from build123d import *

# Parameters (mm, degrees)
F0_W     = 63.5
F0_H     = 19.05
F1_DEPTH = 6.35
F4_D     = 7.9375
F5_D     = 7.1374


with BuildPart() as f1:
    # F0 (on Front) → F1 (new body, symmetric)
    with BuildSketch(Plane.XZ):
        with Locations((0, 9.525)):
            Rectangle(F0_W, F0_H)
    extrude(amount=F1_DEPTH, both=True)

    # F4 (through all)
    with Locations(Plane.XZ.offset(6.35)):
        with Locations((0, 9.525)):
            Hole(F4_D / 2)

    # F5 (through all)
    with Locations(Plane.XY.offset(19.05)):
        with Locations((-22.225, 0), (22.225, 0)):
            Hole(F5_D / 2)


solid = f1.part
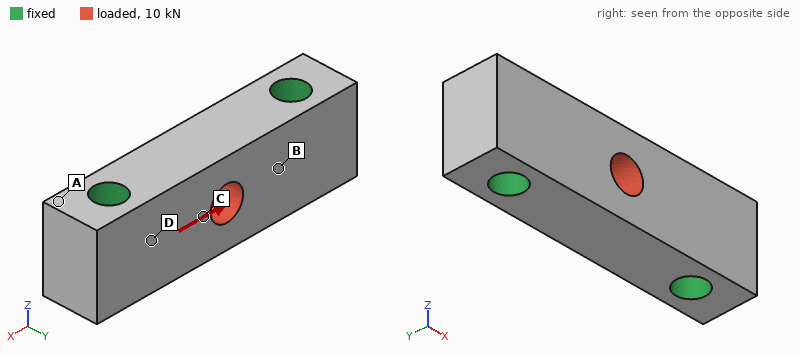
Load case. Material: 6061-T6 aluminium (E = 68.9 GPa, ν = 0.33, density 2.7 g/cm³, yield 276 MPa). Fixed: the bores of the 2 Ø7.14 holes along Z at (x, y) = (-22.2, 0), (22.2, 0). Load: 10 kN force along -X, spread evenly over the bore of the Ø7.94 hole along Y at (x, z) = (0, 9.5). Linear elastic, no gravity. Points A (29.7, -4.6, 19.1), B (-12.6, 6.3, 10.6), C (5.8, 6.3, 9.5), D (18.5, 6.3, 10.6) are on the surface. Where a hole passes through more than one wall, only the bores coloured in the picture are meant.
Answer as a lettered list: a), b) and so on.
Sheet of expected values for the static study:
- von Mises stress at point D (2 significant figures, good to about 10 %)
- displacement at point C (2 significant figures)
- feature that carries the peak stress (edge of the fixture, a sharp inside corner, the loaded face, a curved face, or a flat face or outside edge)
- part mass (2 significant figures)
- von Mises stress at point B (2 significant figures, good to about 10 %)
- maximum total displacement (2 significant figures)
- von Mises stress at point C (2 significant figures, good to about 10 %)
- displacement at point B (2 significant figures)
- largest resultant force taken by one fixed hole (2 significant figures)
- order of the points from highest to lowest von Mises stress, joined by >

a) 11 MPa
b) 5.2 µm
c) the loaded face
d) 36 g
e) 23 MPa
f) 6.8 µm
g) 34 MPa
h) 2.5 µm
i) 5.0 kN
j) C > B > D > A
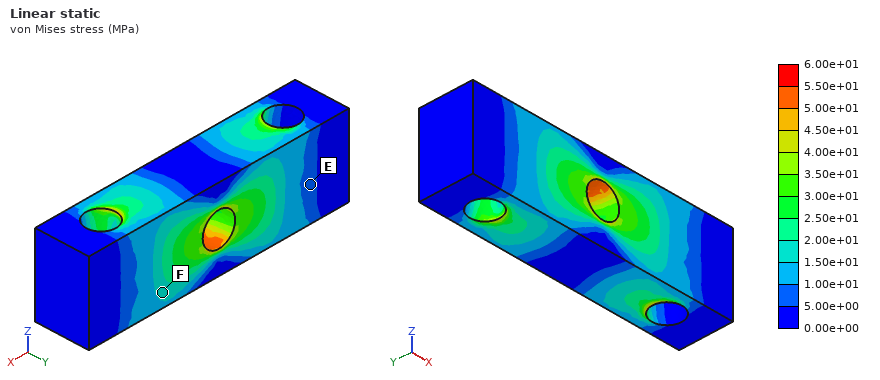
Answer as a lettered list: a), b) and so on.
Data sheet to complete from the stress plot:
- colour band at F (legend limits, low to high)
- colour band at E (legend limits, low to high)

a) 1.50e+01 to 2.00e+01 MPa
b) 5.00e+00 to 1.00e+01 MPa
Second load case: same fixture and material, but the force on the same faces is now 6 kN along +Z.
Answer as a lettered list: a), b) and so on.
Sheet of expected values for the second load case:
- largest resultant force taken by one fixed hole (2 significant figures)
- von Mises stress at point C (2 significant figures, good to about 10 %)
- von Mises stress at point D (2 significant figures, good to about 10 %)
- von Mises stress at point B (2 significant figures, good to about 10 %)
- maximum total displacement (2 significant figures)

a) 3.0 kN
b) 36 MPa
c) 15 MPa
d) 31 MPa
e) 15 µm
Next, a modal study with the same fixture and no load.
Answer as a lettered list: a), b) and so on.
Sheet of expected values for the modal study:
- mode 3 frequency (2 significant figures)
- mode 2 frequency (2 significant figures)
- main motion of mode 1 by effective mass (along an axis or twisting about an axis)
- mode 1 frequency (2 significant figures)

a) 35 kHz
b) 34 kHz
c) along Y
d) 25 kHz
